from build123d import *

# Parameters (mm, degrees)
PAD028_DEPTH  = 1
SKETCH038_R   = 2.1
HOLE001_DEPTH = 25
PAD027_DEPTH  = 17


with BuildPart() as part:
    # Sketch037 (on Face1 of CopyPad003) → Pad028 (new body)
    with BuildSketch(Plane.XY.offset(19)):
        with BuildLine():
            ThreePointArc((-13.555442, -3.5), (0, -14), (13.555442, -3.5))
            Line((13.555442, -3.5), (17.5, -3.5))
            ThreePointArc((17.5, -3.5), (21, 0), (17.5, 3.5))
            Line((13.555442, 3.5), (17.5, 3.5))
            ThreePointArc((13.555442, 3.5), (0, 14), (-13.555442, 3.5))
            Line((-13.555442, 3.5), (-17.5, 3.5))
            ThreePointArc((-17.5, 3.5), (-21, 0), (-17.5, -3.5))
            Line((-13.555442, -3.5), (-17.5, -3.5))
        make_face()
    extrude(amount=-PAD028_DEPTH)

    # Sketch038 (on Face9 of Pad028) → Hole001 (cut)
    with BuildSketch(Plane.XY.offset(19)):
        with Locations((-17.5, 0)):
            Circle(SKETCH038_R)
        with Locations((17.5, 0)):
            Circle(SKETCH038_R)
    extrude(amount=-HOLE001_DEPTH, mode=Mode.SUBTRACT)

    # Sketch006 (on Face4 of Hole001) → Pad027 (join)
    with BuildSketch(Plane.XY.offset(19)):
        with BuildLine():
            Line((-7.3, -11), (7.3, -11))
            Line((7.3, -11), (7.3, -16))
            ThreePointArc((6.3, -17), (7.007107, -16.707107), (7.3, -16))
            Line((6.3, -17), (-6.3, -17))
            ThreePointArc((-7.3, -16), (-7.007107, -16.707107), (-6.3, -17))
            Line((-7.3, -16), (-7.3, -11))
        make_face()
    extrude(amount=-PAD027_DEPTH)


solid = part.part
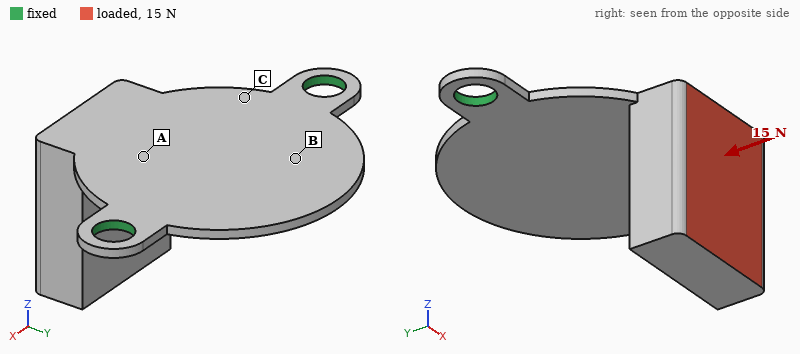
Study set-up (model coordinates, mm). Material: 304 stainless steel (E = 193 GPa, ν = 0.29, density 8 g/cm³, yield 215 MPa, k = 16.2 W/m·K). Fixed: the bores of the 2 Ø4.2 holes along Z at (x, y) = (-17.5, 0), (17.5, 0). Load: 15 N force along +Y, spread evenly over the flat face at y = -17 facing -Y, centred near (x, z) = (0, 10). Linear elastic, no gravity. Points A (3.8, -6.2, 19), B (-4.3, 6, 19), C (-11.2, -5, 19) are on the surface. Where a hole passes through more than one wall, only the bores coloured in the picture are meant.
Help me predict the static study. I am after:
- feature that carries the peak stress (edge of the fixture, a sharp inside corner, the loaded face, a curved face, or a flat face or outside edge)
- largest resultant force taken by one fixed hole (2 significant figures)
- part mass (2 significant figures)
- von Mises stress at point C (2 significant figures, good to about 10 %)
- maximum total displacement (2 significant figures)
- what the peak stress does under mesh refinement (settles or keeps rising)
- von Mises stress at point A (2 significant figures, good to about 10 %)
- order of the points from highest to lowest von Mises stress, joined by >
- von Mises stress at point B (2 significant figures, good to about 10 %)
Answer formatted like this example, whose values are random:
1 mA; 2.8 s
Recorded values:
a sharp inside corner; 7.6 N; 17 g; 35 MPa; 98 µm; keeps rising; 25 MPa; C > A > B; 5.6 MPa
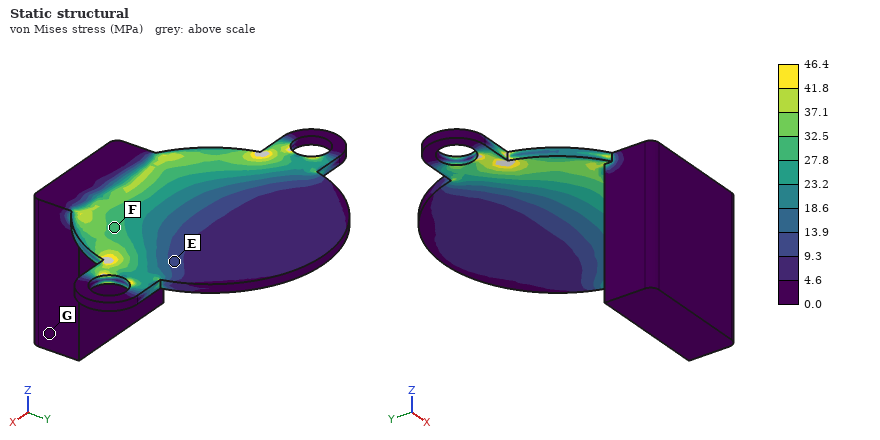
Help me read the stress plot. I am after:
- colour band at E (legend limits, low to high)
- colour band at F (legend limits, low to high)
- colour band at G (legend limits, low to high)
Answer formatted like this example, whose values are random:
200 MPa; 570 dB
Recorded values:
9.3 to 13.9 MPa; 27.8 to 32.5 MPa; 0.0 to 4.6 MPa
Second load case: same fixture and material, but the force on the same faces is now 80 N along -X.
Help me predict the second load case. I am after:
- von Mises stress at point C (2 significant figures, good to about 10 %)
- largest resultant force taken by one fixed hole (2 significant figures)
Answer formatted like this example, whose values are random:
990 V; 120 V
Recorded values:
75 MPa; 65 N
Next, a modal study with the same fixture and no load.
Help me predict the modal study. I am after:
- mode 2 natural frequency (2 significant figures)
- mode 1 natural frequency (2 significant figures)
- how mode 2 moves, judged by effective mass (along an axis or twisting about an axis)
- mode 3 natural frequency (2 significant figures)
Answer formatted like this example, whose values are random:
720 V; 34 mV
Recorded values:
1500 Hz; 530 Hz; along X; 1900 Hz
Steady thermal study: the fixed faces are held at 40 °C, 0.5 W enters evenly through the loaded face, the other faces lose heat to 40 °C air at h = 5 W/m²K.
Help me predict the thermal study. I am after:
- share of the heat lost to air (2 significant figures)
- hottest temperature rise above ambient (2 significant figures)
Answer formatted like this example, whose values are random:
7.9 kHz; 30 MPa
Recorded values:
28 %; 25 K
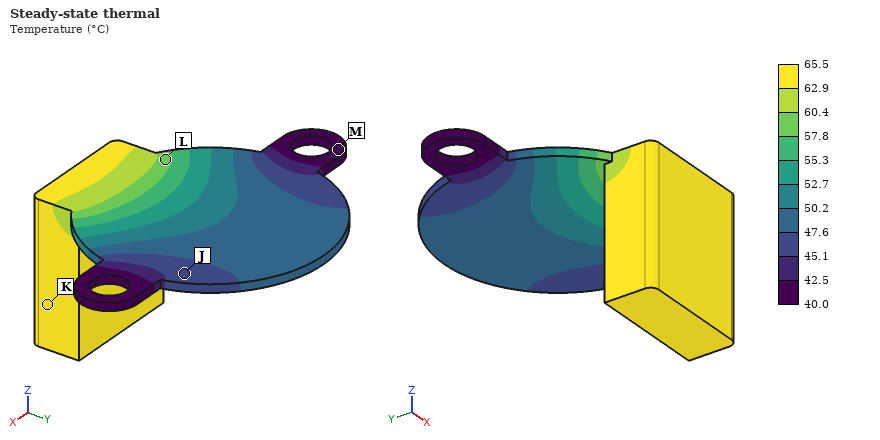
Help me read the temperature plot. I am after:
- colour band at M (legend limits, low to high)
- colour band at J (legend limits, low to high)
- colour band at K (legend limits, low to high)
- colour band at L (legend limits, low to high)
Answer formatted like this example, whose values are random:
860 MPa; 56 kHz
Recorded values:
40.0 to 42.5 °C; 45.1 to 47.6 °C; 62.9 to 65.5 °C; 57.8 to 60.4 °C
